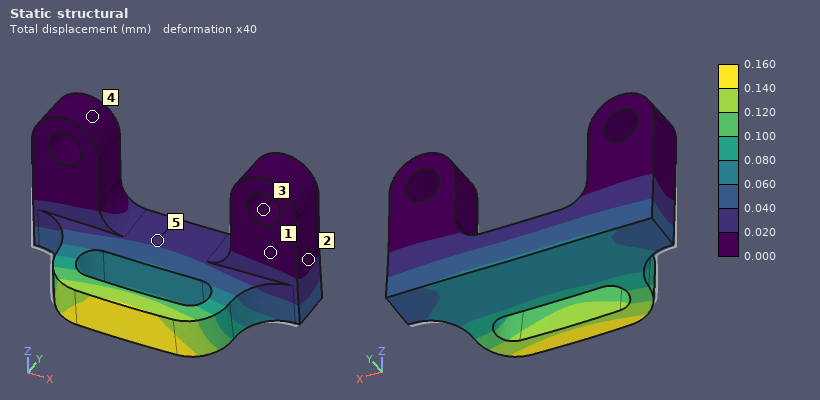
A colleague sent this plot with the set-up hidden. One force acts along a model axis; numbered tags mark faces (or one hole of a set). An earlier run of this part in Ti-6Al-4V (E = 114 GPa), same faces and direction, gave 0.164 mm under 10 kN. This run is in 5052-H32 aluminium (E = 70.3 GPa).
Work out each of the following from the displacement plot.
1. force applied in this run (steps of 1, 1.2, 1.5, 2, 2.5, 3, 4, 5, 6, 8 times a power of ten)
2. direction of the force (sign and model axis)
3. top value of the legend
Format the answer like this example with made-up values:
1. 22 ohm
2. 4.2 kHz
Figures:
1. 6 kN
2. -Z
3. 0.160 mm
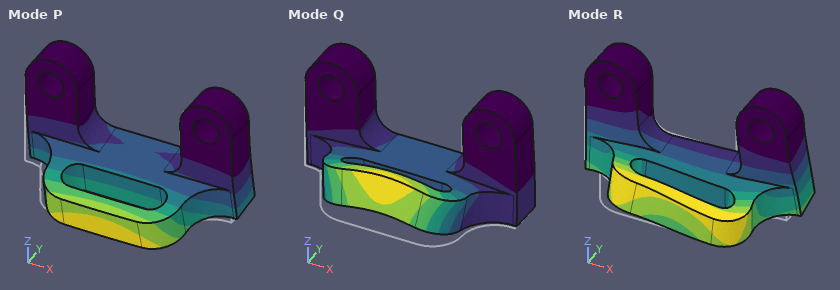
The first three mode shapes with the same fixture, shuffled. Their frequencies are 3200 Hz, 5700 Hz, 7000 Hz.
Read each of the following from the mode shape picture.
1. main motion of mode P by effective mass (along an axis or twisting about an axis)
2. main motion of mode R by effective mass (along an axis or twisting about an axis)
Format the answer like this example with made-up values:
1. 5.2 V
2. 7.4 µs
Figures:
1. along Y
2. along X
